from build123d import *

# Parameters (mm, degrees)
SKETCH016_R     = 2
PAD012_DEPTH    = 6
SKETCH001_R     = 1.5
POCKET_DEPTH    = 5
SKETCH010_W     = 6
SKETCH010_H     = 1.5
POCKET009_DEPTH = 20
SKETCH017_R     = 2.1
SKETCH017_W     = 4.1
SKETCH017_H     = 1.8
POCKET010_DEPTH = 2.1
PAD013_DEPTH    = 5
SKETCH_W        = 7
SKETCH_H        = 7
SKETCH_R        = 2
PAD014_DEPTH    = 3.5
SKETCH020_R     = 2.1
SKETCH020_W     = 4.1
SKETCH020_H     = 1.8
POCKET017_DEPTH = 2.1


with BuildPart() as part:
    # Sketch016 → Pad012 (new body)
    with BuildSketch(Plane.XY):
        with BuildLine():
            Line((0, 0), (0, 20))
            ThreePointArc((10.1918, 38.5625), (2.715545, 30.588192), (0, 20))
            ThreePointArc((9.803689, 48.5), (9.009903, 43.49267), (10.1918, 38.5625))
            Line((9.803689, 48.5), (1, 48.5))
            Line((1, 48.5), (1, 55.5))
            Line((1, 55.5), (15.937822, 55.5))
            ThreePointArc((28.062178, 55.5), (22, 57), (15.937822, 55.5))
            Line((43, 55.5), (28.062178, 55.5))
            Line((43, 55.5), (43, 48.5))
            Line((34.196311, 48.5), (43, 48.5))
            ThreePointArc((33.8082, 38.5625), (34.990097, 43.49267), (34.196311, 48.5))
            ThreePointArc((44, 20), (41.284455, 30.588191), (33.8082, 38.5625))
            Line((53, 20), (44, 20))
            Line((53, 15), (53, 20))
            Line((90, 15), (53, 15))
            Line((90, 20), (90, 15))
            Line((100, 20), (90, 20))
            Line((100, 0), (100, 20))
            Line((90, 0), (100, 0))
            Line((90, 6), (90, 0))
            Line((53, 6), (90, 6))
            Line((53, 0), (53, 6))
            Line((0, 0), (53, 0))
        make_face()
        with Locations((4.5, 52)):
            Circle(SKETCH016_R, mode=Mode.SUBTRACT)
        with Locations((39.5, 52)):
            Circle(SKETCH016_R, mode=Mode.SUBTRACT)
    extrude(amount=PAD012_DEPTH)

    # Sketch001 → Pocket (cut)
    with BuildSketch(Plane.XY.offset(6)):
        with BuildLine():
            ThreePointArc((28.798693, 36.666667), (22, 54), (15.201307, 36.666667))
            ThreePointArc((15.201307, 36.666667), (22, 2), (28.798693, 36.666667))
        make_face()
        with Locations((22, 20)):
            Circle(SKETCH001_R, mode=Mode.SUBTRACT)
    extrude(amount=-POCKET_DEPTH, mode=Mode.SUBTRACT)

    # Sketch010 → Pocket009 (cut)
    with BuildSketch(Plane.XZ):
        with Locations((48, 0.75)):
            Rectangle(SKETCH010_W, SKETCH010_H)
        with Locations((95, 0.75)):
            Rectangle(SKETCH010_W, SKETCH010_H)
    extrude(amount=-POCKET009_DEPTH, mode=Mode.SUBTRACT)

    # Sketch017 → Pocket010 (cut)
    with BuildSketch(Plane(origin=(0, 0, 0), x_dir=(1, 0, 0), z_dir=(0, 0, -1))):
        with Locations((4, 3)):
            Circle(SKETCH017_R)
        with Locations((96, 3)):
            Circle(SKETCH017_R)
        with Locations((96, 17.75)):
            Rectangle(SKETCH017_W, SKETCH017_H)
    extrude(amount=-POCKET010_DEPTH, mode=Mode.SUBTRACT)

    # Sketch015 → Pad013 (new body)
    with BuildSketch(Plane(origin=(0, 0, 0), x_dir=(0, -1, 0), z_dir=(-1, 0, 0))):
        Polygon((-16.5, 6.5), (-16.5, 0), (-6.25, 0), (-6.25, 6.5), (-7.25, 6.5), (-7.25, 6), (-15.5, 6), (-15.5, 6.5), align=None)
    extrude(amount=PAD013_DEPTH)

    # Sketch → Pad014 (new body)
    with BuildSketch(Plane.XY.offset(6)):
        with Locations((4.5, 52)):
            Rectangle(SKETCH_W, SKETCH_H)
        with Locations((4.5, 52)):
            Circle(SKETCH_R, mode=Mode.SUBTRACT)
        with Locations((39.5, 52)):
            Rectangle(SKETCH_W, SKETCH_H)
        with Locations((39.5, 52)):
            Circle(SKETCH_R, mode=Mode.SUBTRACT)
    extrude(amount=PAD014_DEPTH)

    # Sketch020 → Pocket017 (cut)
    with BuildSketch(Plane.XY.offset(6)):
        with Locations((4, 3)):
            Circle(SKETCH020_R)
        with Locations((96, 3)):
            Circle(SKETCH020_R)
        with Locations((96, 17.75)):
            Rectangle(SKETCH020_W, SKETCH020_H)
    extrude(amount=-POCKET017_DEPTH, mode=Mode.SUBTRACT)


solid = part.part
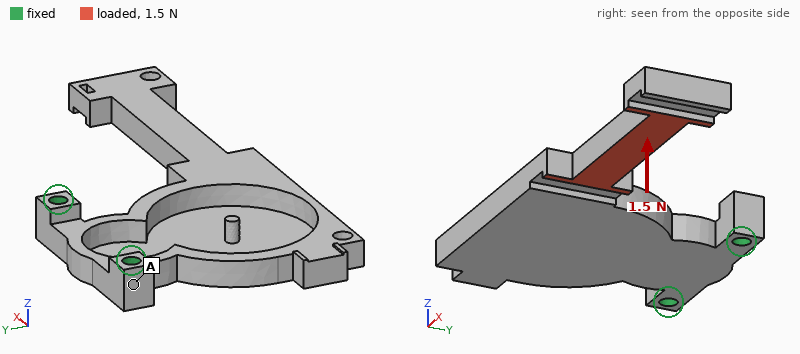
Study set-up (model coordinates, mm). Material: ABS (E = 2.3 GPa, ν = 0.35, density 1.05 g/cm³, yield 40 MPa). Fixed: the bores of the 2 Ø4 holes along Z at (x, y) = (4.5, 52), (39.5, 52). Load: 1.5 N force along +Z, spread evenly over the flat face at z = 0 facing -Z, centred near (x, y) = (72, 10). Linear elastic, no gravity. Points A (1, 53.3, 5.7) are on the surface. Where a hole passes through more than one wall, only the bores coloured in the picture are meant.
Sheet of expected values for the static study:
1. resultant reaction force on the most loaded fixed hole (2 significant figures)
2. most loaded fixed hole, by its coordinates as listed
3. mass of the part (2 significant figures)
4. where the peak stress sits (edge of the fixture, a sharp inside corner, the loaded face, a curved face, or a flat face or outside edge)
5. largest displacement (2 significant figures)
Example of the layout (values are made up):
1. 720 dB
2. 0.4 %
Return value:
1. 3.8 N
2. (39.5, 52)
3. 11 g
4. a curved face
5. 1.1 mm
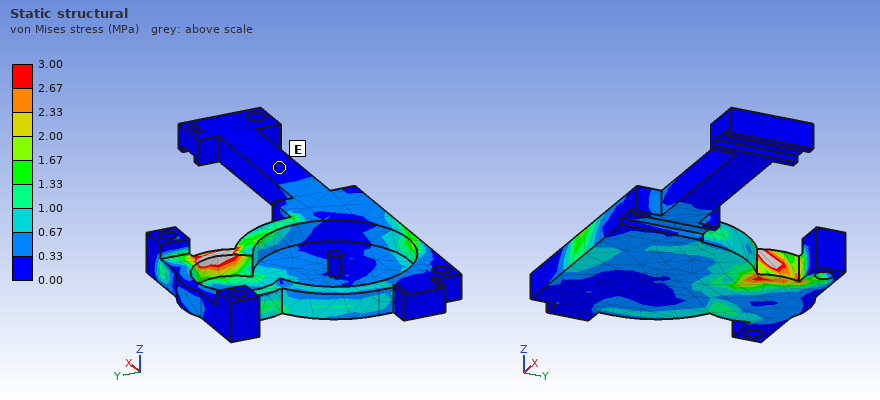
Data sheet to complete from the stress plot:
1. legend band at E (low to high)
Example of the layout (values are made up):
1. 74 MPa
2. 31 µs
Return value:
1. 0.00 to 0.33 MPa
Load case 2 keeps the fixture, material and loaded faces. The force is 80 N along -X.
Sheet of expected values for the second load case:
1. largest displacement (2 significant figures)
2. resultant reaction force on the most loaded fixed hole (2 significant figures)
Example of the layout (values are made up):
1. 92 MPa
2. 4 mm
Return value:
1. 1.2 mm
2. 130 N
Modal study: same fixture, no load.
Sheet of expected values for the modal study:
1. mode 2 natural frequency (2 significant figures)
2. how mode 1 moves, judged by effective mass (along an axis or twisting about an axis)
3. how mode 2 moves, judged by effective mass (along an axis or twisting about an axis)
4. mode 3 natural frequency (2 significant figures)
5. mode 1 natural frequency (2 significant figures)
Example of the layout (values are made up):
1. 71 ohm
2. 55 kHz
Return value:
1. 260 Hz
2. along Z
3. along Z
4. 420 Hz
5. 110 Hz
